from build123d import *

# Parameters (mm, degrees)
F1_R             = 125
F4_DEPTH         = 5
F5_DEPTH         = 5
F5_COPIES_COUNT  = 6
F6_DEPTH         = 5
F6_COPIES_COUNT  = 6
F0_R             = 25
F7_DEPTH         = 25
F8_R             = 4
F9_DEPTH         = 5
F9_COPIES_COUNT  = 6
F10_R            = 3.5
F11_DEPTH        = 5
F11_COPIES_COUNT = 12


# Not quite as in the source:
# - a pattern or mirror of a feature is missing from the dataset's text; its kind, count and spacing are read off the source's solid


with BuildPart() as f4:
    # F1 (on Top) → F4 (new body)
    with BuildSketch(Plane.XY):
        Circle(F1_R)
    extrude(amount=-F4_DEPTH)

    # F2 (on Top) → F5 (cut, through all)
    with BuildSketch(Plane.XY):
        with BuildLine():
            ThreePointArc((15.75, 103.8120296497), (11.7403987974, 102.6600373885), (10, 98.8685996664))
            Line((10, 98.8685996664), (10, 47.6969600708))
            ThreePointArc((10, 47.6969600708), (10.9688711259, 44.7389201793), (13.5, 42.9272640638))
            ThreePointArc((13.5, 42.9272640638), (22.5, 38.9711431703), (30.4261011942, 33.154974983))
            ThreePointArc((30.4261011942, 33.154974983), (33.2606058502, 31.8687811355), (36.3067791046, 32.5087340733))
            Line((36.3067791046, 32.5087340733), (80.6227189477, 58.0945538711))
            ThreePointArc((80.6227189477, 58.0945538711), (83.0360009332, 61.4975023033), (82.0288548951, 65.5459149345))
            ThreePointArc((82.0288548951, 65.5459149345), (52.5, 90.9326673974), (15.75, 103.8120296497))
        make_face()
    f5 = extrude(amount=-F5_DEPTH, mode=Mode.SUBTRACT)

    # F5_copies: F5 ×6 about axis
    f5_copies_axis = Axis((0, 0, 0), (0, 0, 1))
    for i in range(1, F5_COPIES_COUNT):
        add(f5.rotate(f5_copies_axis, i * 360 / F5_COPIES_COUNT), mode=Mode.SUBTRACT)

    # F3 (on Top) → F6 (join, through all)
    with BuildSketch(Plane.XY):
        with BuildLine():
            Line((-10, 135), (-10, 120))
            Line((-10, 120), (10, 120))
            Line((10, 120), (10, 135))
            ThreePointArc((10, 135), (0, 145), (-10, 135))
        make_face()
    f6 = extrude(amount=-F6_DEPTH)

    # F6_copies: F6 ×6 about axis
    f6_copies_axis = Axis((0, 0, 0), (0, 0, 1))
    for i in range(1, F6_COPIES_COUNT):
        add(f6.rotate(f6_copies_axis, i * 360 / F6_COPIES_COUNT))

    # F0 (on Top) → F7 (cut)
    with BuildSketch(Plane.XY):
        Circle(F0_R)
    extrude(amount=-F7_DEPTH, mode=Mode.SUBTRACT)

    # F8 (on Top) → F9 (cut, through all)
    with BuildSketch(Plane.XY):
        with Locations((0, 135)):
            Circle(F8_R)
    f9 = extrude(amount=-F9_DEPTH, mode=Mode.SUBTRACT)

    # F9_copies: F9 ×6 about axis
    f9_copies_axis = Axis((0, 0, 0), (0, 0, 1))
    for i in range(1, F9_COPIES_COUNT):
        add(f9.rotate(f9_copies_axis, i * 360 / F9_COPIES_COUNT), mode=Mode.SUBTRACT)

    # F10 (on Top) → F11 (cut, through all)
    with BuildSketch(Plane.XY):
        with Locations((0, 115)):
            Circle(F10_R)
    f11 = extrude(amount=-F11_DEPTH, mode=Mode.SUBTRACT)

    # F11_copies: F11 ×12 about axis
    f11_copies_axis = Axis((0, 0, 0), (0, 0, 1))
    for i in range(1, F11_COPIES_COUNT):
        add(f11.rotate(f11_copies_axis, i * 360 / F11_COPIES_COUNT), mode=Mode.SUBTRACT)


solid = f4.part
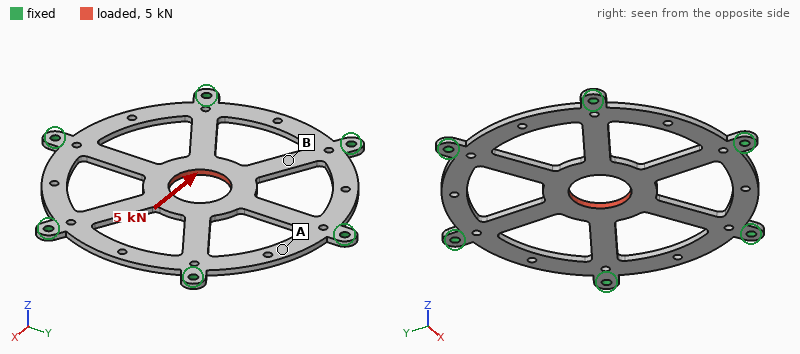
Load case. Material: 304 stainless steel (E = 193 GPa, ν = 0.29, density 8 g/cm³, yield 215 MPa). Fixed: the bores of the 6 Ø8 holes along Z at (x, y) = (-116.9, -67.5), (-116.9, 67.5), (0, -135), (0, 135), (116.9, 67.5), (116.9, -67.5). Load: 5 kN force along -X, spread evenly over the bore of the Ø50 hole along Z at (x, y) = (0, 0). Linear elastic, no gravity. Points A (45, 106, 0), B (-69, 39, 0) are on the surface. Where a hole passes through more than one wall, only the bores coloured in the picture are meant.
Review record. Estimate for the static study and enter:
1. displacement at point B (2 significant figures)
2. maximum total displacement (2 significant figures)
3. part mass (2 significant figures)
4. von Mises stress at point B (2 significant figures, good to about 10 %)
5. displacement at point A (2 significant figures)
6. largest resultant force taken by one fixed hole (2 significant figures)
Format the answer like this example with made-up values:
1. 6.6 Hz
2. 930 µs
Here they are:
1. 4.6 µm
2. 9.1 µm
3. 1.1 kg
4. 14 MPa
5. 1.5 µm
6. 1.3 kN
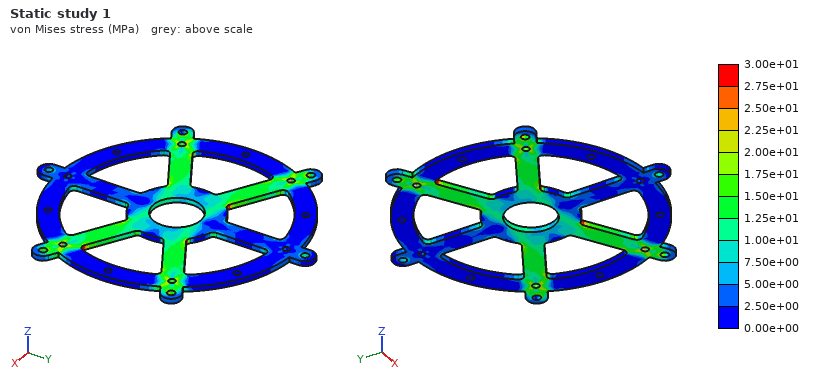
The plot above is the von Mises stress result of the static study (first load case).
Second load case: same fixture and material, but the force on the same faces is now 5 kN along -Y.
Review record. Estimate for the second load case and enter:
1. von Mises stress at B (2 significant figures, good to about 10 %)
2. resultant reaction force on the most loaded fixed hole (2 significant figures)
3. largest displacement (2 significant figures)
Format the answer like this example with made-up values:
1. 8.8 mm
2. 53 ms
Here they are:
1. 8.1 MPa
2. 1.5 kN
3. 9.0 µm
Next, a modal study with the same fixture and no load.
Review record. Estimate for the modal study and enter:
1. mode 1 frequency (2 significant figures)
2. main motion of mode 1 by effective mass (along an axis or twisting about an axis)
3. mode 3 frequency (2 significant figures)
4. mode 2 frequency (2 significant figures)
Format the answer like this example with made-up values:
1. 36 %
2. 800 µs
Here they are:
1. 450 Hz
2. along Z
3. 1000 Hz
4. 1000 Hz
